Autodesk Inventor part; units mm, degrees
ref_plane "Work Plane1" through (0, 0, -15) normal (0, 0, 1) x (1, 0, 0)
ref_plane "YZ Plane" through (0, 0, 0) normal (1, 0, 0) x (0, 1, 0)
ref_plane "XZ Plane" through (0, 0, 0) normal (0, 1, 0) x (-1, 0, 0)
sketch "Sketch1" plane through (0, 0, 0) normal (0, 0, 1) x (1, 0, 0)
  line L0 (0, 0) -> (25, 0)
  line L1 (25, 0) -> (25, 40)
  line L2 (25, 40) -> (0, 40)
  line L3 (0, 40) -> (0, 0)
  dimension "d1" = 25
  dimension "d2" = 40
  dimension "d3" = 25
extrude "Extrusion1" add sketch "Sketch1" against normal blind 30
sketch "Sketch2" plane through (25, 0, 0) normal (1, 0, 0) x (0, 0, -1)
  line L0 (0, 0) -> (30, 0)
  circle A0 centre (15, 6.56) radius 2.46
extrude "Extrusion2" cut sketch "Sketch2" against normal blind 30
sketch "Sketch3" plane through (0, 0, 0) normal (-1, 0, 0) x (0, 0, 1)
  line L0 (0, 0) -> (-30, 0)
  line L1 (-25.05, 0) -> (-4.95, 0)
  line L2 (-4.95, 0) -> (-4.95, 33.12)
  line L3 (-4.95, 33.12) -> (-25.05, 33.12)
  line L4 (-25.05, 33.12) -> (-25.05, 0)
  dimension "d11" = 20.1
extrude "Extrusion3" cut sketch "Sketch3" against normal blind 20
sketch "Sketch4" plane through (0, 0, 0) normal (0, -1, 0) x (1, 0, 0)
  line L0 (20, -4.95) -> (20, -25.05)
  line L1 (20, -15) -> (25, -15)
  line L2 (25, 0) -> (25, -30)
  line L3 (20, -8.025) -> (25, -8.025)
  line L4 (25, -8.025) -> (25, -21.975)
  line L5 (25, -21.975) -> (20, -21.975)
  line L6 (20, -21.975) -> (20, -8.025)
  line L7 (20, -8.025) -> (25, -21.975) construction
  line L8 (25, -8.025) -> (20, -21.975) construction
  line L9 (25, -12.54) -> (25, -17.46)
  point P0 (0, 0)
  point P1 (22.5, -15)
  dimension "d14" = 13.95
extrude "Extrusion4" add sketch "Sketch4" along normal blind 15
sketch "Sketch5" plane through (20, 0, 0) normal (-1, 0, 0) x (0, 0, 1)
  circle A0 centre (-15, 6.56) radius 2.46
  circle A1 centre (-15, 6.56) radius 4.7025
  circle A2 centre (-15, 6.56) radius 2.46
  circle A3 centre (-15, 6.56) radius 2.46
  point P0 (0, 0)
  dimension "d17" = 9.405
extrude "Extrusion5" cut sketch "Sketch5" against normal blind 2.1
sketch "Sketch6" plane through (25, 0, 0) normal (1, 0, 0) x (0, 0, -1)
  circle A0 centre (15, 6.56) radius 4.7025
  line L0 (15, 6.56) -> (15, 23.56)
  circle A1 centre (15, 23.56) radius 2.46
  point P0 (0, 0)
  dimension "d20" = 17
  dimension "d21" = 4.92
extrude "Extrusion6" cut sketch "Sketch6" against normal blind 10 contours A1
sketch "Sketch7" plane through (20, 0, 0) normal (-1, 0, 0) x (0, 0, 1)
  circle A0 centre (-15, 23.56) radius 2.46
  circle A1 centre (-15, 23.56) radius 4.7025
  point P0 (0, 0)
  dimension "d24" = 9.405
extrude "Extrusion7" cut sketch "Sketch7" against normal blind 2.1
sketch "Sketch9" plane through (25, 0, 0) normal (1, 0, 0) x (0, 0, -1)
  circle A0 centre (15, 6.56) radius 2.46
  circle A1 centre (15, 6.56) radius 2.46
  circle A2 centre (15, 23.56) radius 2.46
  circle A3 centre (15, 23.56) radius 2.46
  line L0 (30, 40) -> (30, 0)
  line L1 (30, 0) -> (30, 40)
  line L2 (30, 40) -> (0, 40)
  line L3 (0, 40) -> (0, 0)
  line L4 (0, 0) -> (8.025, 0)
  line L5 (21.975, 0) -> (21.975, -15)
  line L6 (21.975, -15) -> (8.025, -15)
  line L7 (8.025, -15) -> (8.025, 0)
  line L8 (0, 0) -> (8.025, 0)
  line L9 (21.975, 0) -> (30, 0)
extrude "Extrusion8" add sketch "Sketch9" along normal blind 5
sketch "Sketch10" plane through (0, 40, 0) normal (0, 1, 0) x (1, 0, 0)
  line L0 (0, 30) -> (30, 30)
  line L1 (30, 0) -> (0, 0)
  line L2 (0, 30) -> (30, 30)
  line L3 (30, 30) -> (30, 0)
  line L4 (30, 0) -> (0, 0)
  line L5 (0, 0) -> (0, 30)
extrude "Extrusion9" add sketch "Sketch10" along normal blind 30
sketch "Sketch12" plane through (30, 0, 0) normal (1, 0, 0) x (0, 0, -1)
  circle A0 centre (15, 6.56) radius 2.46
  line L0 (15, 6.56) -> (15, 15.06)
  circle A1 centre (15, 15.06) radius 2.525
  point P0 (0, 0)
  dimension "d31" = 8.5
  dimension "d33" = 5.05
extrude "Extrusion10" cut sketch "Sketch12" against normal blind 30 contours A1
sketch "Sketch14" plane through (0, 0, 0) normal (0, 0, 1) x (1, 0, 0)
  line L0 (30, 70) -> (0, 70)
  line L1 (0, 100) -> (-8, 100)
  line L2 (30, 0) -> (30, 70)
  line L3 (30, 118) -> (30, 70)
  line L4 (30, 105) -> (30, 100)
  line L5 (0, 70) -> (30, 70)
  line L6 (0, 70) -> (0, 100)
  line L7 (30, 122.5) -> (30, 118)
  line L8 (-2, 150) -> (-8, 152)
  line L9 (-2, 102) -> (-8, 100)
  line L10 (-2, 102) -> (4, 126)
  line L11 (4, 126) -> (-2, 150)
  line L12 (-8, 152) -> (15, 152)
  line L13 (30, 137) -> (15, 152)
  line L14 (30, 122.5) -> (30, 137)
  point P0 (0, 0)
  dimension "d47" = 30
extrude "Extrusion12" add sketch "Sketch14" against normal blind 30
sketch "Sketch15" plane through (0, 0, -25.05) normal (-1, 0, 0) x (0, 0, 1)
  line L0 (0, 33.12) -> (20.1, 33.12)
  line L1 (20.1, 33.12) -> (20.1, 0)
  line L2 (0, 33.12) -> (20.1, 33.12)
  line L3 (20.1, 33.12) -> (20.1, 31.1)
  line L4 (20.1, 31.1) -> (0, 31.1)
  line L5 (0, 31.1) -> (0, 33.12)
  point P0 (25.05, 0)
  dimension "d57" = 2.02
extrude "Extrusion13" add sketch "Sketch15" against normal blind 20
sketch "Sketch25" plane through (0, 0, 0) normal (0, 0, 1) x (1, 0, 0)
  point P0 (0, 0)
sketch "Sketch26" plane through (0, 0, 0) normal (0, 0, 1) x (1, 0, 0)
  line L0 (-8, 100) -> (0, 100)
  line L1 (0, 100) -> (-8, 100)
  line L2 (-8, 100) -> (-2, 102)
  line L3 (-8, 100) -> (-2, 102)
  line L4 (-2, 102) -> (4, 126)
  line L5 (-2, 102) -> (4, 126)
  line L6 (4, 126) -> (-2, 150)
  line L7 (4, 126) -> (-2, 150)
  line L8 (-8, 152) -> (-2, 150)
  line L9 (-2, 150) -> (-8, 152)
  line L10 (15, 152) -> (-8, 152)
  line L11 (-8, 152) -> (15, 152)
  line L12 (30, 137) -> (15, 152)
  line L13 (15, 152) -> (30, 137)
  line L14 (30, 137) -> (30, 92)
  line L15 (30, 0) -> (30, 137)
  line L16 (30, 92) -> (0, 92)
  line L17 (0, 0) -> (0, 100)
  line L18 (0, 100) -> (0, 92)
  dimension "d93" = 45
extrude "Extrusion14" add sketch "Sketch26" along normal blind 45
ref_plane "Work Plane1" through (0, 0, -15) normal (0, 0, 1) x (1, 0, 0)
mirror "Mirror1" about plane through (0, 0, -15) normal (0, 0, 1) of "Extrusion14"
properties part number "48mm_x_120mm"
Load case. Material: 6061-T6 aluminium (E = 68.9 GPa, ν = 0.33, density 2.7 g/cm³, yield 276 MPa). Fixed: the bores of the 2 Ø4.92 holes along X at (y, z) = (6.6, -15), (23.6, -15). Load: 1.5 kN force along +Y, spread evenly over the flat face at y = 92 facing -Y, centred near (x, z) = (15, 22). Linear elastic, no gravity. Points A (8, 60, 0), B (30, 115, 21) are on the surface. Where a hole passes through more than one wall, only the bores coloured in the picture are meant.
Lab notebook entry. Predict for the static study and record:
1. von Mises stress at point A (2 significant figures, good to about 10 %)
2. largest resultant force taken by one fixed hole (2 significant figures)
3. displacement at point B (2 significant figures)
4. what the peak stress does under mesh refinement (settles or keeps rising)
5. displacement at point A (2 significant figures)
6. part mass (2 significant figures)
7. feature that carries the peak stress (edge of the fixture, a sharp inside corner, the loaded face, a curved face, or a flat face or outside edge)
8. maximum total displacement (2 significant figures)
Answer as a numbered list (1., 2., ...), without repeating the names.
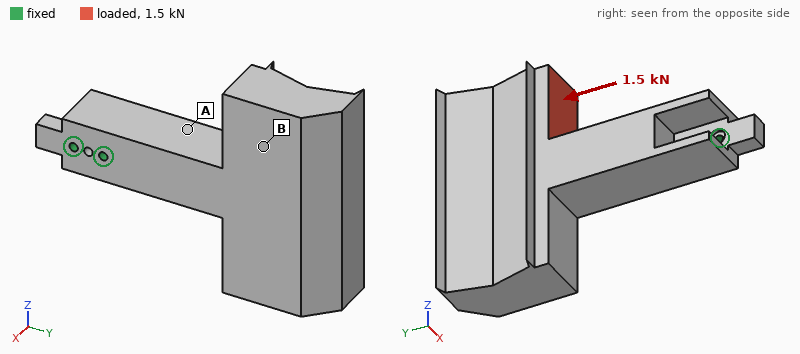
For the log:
1. 13 MPa
2. 2.7 kN
3. 0.15 mm
4. keeps rising
5. 0.044 mm
6. 730 g
7. edge of the fixture
8. 0.23 mm
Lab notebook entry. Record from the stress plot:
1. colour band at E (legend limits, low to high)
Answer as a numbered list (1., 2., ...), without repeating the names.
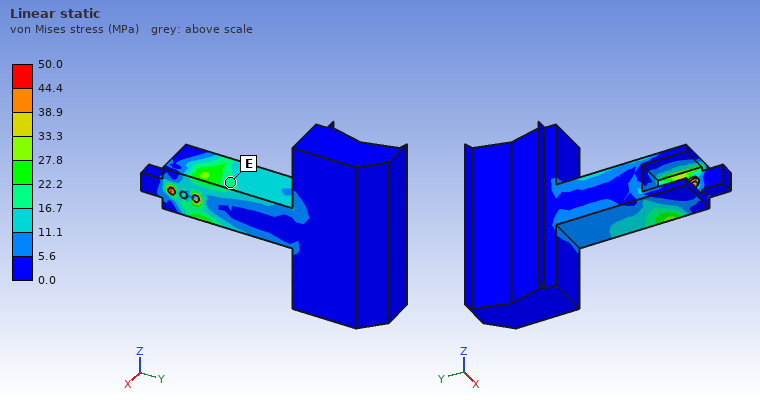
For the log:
1. 16.7 to 22.2 MPa
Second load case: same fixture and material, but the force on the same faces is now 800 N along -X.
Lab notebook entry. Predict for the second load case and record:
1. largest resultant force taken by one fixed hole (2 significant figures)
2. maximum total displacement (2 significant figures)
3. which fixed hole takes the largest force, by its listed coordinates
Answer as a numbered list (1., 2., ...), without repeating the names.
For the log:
1. 2.9 kN
2. 0.32 mm
3. (23.6, -15)
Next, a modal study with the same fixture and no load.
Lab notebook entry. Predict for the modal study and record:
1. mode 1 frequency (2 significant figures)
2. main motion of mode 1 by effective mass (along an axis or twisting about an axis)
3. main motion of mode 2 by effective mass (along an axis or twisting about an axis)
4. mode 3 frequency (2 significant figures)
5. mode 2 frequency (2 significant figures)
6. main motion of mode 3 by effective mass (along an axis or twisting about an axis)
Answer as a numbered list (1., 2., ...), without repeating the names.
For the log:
1. 400 Hz
2. along X
3. along Z
4. 720 Hz
5. 440 Hz
6. twisting about Y
